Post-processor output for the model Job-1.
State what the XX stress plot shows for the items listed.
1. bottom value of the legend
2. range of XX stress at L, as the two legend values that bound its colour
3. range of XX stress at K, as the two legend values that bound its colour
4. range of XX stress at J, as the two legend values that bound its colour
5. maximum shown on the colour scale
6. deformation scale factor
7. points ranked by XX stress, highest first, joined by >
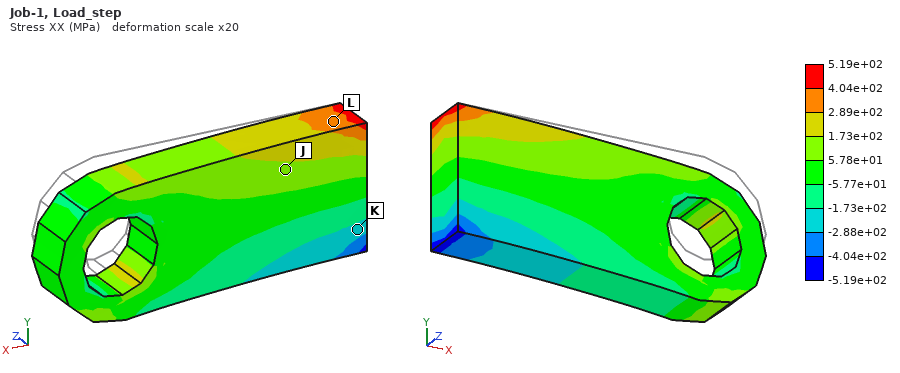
-5.19e+02 MPa
2.89e+02 to 4.04e+02 MPa
-2.88e+02 to -1.73e+02 MPa
5.78e+01 to 1.73e+02 MPa
5.19e+02 MPa
20
L > J > K
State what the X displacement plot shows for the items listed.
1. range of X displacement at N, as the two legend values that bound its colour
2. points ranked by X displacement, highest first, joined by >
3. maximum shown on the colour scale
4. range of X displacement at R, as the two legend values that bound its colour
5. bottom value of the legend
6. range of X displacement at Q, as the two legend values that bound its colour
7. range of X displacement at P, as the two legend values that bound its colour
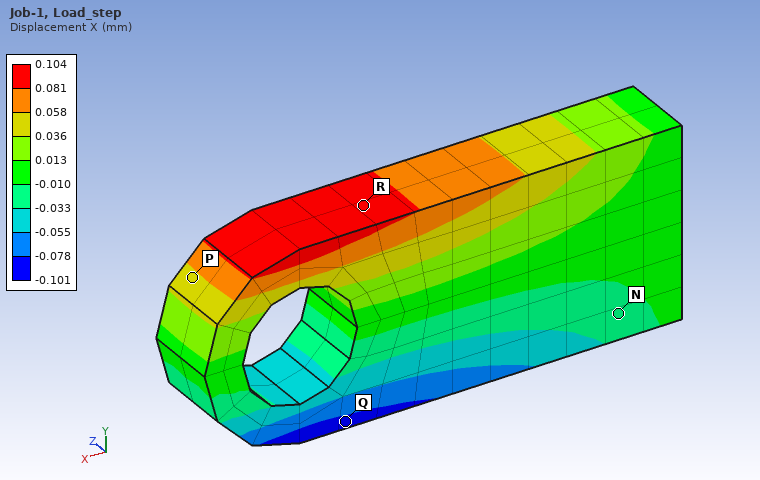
-0.033 to -0.010 mm
R > P > N > Q
0.104 mm
0.081 to 0.104 mm
-0.101 mm
-0.101 to -0.078 mm
0.036 to 0.058 mm
